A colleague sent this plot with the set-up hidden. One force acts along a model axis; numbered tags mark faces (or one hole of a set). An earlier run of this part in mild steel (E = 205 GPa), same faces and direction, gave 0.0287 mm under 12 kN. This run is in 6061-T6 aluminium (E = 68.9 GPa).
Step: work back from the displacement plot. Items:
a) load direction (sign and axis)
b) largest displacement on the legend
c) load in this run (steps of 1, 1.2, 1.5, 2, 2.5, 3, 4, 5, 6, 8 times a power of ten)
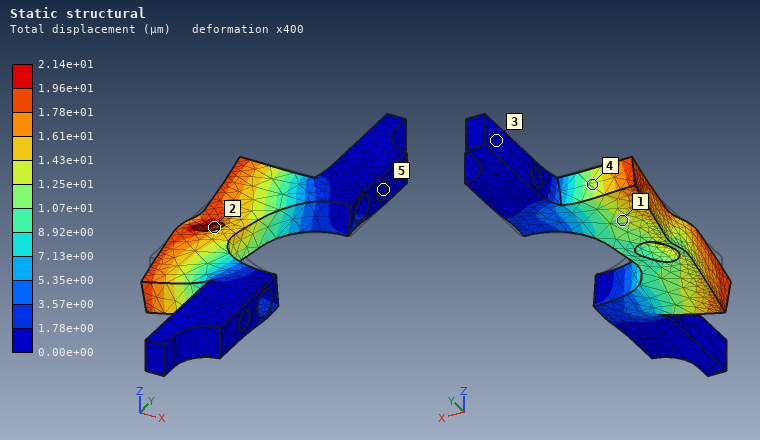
-Y
2.14e+01 µm
3 kN
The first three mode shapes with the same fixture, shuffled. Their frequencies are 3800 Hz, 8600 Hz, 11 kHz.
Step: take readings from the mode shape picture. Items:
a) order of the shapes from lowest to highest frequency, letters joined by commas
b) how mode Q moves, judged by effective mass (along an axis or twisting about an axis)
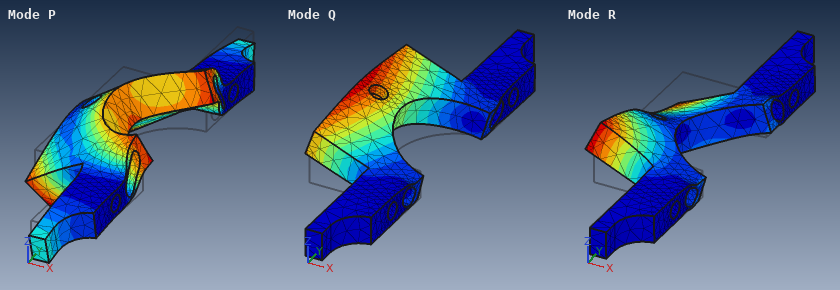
Q, R, P
along Z
